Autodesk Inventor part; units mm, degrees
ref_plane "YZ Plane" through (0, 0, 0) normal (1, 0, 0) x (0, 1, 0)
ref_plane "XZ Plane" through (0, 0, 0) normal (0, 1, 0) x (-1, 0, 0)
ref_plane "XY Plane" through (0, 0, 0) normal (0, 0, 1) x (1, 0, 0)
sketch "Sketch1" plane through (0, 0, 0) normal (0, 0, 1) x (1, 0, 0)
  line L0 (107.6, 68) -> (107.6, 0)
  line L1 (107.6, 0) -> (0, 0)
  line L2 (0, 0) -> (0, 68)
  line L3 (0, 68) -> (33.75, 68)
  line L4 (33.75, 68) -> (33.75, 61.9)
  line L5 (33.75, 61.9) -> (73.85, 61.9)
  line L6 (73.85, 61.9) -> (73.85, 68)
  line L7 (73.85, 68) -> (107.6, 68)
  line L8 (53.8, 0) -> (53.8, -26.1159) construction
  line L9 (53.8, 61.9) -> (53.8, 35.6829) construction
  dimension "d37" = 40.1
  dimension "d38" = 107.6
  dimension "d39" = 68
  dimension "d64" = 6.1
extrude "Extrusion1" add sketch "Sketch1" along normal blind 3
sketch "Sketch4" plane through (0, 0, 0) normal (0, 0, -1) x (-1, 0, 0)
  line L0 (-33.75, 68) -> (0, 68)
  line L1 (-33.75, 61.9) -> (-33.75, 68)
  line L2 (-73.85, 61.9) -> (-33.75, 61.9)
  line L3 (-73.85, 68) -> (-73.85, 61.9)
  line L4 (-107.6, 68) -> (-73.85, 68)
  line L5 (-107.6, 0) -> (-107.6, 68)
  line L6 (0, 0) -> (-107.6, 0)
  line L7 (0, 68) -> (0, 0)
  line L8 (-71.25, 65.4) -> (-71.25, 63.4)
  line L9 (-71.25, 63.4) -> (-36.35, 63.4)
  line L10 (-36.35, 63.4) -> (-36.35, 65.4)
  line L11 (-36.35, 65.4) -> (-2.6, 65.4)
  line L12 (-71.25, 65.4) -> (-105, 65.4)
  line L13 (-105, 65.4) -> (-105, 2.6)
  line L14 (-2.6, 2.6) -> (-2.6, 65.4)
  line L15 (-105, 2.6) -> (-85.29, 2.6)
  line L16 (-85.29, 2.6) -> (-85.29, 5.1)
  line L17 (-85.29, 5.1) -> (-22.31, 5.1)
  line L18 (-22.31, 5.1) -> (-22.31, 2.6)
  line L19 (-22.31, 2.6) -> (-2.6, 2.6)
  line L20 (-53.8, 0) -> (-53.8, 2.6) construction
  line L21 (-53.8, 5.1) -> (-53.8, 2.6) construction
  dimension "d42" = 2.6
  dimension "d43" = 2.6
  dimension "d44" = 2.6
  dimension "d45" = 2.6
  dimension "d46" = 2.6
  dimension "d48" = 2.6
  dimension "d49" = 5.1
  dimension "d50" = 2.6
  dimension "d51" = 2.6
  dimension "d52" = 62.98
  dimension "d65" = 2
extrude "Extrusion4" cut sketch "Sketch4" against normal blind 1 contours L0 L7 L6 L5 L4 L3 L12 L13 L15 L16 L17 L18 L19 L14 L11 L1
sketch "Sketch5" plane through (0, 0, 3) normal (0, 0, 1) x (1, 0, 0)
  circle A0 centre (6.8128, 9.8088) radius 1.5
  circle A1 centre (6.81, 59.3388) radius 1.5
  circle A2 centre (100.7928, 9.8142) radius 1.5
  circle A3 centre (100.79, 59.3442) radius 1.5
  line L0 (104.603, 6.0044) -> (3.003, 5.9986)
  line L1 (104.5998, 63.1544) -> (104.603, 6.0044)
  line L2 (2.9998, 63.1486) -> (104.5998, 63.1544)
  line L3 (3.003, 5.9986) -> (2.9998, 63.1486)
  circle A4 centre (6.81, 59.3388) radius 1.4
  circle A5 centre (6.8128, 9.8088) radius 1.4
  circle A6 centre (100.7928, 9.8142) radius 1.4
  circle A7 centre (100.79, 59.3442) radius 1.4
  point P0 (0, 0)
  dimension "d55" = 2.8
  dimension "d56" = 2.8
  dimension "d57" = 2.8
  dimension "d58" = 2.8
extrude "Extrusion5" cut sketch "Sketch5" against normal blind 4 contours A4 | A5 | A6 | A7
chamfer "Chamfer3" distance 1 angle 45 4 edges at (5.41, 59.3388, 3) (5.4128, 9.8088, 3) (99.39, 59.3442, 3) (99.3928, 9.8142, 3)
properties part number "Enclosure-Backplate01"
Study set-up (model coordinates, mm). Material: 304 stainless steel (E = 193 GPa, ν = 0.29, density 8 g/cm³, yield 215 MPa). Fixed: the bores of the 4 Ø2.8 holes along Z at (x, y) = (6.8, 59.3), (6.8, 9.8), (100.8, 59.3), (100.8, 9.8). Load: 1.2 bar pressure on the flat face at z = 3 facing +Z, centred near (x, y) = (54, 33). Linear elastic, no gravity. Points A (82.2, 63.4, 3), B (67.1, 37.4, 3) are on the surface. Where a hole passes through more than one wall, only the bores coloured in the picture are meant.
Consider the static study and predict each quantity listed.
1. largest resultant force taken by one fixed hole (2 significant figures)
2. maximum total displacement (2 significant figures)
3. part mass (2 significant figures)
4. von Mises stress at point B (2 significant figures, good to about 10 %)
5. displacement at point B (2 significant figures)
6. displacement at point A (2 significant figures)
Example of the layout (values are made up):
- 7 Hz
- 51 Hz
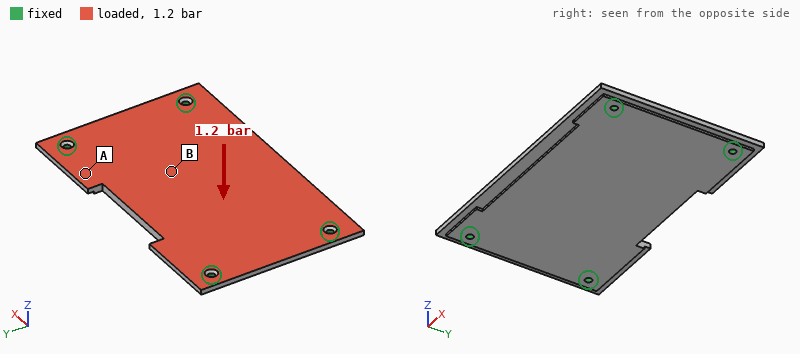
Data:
- 280 N
- 97 µm
- 160 g
- 28 MPa
- 80 µm
- 38 µm
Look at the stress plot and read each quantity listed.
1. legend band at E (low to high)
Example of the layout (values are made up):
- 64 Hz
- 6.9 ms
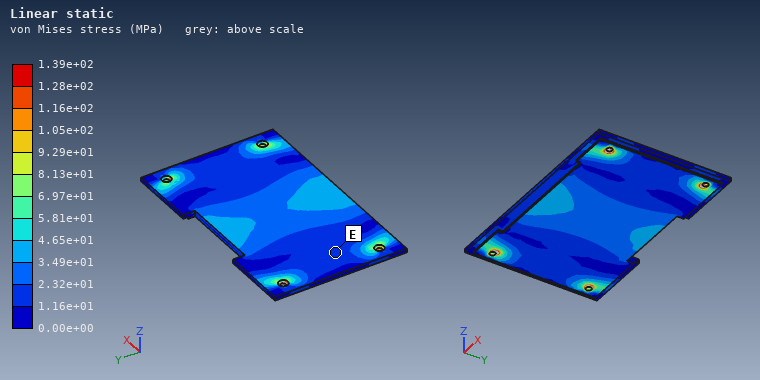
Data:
- 1.16e+01 to 2.32e+01 MPa
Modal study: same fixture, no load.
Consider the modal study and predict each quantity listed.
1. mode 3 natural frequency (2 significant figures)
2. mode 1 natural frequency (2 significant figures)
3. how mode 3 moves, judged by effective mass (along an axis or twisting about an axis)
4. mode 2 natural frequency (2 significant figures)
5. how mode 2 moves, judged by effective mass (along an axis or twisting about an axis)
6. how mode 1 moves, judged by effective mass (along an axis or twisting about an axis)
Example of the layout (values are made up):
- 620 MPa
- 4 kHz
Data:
- 3700 Hz
- 1400 Hz
- twisting about Y
- 2300 Hz
- twisting about X
- along Z
